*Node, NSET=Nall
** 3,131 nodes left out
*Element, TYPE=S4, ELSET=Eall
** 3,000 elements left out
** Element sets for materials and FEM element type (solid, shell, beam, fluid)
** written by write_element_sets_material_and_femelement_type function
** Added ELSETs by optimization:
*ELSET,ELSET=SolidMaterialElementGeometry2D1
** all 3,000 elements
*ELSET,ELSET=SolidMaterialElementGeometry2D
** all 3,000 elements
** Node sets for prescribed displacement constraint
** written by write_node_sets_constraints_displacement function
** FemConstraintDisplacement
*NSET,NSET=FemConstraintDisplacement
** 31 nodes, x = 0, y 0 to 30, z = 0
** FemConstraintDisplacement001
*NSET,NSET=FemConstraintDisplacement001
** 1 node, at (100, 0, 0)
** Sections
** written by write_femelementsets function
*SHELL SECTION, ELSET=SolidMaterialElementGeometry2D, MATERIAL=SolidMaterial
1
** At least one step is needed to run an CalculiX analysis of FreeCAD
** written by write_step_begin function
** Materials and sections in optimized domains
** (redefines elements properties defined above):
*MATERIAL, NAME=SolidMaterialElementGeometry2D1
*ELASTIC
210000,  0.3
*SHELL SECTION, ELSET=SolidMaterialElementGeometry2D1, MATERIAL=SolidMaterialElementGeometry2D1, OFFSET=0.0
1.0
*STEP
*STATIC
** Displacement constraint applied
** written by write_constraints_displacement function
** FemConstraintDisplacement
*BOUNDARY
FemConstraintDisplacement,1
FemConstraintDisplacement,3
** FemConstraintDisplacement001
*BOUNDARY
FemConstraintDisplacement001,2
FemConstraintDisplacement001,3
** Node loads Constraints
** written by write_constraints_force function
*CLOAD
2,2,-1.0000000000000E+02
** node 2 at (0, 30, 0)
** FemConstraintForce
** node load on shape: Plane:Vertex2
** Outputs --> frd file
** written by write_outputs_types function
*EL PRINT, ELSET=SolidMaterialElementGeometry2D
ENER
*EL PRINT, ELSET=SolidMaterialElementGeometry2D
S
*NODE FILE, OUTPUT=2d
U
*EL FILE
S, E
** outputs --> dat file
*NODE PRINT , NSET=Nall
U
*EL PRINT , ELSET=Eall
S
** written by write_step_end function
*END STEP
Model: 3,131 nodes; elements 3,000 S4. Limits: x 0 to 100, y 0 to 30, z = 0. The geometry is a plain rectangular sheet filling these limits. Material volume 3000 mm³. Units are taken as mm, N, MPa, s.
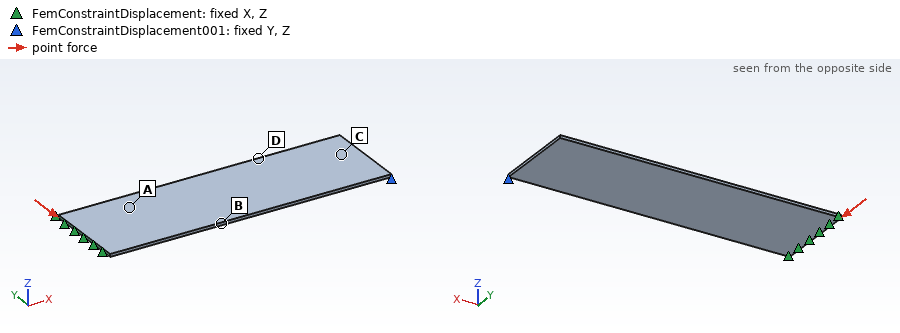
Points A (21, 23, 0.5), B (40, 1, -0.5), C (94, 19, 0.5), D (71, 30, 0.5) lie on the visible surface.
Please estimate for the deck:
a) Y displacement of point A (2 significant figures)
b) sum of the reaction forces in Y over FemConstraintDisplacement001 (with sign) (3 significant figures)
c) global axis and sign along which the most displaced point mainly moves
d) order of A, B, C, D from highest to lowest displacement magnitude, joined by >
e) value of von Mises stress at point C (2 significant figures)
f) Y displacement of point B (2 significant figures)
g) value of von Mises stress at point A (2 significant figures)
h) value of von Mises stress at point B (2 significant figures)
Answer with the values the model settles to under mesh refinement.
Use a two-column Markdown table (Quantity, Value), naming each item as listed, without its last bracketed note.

| Quantity | Value |
|---|---|
| Y displacement of point A | -0.074 mm |
| sum of the reaction forces in Y over FemConstraintDisplacement001 (with sign) | 100 N |
| global axis and sign along which the most displaced point mainly moves | -Y |
| order of A, B, C, D from highest to lowest displacement magnitude, joined by > | A > B > D > C |
| value of von Mises stress at point C | 8.1 MPa |
| Y displacement of point B | -0.063 mm |
| value of von Mises stress at point A | 29 MPa |
| value of von Mises stress at point B | 37 MPa |
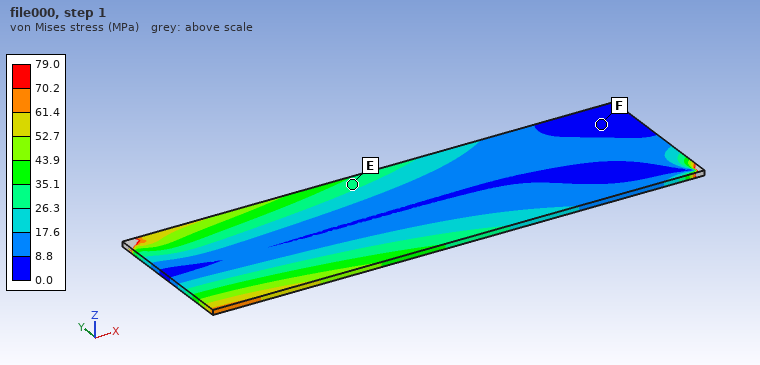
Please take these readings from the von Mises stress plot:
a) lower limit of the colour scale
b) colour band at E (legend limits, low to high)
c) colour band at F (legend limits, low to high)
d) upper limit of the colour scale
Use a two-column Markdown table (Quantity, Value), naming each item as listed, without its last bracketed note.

| Quantity | Value |
|---|---|
| lower limit of the colour scale | 0.0 MPa |
| colour band at E | 26.3 to 35.1 MPa |
| colour band at F | 0.0 to 8.8 MPa |
| upper limit of the colour scale | 79.0 MPa |
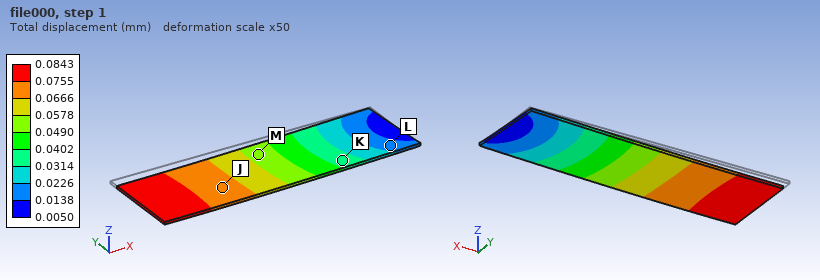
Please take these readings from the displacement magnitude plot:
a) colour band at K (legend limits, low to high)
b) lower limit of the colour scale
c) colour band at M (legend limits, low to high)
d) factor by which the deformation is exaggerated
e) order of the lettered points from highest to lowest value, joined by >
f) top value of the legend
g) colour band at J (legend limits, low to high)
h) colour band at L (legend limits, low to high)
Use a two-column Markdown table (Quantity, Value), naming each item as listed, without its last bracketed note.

| Quantity | Value |
|---|---|
| colour band at K | 0.0314 to 0.0402 mm |
| lower limit of the colour scale | 0.0050 mm |
| colour band at M | 0.0490 to 0.0578 mm |
| factor by which the deformation is exaggerated | 50 |
| order of the lettered points from highest to lowest value, joined by > | J > M > K > L |
| top value of the legend | 0.0843 mm |
| colour band at J | 0.0666 to 0.0755 mm |
| colour band at L | 0.0138 to 0.0226 mm |
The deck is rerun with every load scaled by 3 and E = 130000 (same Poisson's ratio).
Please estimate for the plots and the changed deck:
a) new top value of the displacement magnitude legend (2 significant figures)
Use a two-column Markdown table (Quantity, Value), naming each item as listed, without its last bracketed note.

| Quantity | Value |
|---|---|
| new top value of the displacement magnitude legend | 0.41 mm |
